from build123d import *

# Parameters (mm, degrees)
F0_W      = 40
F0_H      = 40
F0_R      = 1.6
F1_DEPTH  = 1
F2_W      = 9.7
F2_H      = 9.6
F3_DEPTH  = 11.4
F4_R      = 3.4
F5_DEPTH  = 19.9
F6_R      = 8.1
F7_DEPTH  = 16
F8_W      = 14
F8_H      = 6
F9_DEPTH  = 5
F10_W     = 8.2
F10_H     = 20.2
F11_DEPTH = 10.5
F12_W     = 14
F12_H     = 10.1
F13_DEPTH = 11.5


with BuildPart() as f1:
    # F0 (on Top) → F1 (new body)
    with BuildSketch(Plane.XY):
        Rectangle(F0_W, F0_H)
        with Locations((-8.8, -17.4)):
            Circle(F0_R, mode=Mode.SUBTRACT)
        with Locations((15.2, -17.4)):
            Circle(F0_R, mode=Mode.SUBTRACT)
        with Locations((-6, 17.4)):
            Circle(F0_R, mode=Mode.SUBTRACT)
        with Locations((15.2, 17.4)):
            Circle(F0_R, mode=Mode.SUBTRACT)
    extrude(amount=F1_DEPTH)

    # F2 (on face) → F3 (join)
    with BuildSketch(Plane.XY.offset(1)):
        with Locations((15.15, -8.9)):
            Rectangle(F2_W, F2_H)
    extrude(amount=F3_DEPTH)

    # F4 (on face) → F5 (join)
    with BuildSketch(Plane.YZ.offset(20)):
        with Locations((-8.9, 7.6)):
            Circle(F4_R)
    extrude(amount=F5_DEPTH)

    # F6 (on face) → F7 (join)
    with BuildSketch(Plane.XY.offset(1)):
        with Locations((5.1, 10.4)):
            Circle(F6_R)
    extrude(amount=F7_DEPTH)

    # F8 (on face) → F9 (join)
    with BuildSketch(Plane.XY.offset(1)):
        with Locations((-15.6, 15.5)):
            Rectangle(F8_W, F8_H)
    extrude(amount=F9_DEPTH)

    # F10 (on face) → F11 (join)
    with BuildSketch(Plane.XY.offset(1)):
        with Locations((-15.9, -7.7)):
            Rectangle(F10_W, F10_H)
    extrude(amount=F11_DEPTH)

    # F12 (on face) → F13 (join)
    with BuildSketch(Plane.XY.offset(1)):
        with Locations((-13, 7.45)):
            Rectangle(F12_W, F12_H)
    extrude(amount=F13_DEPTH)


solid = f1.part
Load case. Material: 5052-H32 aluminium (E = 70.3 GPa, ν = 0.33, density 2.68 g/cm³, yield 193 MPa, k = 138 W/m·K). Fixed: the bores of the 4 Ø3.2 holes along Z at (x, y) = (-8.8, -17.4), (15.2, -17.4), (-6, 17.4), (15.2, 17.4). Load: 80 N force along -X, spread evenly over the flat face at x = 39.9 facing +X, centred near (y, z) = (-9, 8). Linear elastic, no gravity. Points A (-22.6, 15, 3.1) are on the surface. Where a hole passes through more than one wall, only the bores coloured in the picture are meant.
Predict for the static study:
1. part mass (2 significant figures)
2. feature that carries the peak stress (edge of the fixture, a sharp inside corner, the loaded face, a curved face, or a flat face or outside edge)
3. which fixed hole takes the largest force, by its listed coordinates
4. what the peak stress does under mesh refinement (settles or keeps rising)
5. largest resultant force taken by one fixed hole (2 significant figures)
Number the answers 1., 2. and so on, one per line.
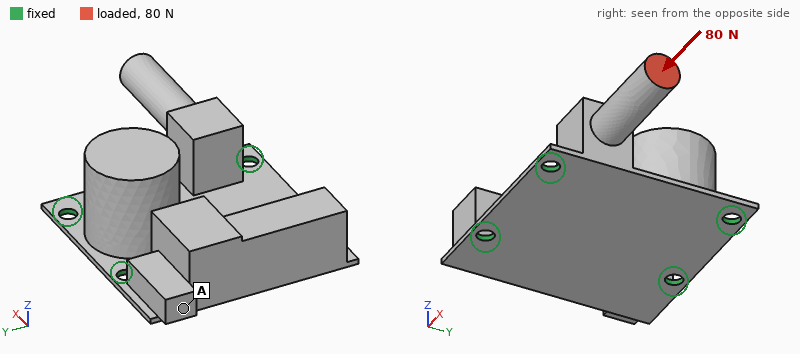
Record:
1. 28 g
2. edge of the fixture
3. (15.2, -17.4)
4. keeps rising
5. 40 N
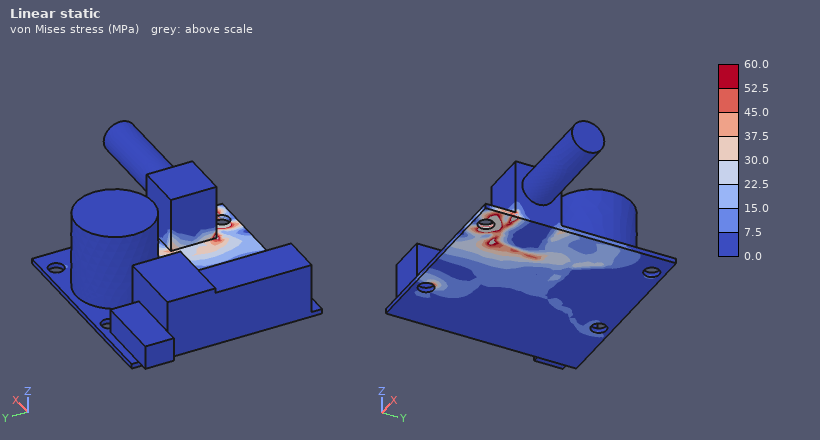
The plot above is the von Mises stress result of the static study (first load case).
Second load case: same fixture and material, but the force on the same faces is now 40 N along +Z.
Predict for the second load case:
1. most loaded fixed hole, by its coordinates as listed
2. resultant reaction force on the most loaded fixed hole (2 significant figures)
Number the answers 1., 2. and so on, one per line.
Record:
1. (15.2, -17.4)
2. 52 N
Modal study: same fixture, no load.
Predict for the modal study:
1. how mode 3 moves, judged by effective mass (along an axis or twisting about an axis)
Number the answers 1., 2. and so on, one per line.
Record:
1. along Z
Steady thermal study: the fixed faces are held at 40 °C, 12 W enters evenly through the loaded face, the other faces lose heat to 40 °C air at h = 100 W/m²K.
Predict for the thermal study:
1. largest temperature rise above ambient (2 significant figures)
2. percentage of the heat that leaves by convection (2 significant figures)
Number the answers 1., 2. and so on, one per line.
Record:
1. 67 K
2. 36 %
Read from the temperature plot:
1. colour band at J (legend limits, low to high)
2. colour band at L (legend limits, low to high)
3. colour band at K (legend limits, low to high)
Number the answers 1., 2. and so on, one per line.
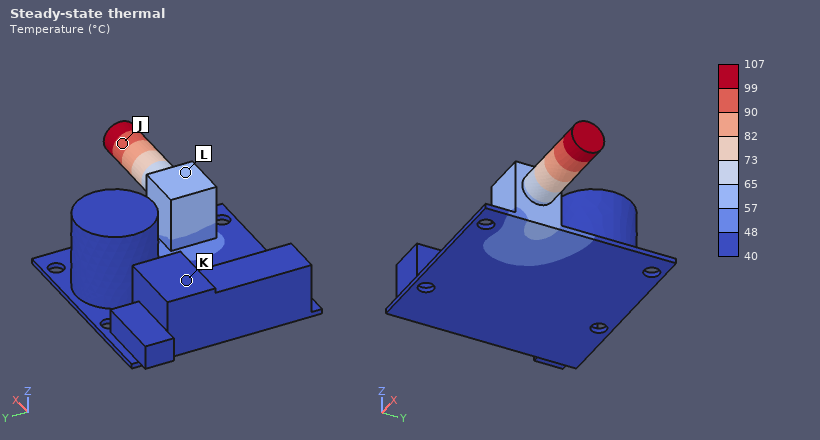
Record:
1. 90 to 99 °C
2. 57 to 65 °C
3. 40 to 48 °C
